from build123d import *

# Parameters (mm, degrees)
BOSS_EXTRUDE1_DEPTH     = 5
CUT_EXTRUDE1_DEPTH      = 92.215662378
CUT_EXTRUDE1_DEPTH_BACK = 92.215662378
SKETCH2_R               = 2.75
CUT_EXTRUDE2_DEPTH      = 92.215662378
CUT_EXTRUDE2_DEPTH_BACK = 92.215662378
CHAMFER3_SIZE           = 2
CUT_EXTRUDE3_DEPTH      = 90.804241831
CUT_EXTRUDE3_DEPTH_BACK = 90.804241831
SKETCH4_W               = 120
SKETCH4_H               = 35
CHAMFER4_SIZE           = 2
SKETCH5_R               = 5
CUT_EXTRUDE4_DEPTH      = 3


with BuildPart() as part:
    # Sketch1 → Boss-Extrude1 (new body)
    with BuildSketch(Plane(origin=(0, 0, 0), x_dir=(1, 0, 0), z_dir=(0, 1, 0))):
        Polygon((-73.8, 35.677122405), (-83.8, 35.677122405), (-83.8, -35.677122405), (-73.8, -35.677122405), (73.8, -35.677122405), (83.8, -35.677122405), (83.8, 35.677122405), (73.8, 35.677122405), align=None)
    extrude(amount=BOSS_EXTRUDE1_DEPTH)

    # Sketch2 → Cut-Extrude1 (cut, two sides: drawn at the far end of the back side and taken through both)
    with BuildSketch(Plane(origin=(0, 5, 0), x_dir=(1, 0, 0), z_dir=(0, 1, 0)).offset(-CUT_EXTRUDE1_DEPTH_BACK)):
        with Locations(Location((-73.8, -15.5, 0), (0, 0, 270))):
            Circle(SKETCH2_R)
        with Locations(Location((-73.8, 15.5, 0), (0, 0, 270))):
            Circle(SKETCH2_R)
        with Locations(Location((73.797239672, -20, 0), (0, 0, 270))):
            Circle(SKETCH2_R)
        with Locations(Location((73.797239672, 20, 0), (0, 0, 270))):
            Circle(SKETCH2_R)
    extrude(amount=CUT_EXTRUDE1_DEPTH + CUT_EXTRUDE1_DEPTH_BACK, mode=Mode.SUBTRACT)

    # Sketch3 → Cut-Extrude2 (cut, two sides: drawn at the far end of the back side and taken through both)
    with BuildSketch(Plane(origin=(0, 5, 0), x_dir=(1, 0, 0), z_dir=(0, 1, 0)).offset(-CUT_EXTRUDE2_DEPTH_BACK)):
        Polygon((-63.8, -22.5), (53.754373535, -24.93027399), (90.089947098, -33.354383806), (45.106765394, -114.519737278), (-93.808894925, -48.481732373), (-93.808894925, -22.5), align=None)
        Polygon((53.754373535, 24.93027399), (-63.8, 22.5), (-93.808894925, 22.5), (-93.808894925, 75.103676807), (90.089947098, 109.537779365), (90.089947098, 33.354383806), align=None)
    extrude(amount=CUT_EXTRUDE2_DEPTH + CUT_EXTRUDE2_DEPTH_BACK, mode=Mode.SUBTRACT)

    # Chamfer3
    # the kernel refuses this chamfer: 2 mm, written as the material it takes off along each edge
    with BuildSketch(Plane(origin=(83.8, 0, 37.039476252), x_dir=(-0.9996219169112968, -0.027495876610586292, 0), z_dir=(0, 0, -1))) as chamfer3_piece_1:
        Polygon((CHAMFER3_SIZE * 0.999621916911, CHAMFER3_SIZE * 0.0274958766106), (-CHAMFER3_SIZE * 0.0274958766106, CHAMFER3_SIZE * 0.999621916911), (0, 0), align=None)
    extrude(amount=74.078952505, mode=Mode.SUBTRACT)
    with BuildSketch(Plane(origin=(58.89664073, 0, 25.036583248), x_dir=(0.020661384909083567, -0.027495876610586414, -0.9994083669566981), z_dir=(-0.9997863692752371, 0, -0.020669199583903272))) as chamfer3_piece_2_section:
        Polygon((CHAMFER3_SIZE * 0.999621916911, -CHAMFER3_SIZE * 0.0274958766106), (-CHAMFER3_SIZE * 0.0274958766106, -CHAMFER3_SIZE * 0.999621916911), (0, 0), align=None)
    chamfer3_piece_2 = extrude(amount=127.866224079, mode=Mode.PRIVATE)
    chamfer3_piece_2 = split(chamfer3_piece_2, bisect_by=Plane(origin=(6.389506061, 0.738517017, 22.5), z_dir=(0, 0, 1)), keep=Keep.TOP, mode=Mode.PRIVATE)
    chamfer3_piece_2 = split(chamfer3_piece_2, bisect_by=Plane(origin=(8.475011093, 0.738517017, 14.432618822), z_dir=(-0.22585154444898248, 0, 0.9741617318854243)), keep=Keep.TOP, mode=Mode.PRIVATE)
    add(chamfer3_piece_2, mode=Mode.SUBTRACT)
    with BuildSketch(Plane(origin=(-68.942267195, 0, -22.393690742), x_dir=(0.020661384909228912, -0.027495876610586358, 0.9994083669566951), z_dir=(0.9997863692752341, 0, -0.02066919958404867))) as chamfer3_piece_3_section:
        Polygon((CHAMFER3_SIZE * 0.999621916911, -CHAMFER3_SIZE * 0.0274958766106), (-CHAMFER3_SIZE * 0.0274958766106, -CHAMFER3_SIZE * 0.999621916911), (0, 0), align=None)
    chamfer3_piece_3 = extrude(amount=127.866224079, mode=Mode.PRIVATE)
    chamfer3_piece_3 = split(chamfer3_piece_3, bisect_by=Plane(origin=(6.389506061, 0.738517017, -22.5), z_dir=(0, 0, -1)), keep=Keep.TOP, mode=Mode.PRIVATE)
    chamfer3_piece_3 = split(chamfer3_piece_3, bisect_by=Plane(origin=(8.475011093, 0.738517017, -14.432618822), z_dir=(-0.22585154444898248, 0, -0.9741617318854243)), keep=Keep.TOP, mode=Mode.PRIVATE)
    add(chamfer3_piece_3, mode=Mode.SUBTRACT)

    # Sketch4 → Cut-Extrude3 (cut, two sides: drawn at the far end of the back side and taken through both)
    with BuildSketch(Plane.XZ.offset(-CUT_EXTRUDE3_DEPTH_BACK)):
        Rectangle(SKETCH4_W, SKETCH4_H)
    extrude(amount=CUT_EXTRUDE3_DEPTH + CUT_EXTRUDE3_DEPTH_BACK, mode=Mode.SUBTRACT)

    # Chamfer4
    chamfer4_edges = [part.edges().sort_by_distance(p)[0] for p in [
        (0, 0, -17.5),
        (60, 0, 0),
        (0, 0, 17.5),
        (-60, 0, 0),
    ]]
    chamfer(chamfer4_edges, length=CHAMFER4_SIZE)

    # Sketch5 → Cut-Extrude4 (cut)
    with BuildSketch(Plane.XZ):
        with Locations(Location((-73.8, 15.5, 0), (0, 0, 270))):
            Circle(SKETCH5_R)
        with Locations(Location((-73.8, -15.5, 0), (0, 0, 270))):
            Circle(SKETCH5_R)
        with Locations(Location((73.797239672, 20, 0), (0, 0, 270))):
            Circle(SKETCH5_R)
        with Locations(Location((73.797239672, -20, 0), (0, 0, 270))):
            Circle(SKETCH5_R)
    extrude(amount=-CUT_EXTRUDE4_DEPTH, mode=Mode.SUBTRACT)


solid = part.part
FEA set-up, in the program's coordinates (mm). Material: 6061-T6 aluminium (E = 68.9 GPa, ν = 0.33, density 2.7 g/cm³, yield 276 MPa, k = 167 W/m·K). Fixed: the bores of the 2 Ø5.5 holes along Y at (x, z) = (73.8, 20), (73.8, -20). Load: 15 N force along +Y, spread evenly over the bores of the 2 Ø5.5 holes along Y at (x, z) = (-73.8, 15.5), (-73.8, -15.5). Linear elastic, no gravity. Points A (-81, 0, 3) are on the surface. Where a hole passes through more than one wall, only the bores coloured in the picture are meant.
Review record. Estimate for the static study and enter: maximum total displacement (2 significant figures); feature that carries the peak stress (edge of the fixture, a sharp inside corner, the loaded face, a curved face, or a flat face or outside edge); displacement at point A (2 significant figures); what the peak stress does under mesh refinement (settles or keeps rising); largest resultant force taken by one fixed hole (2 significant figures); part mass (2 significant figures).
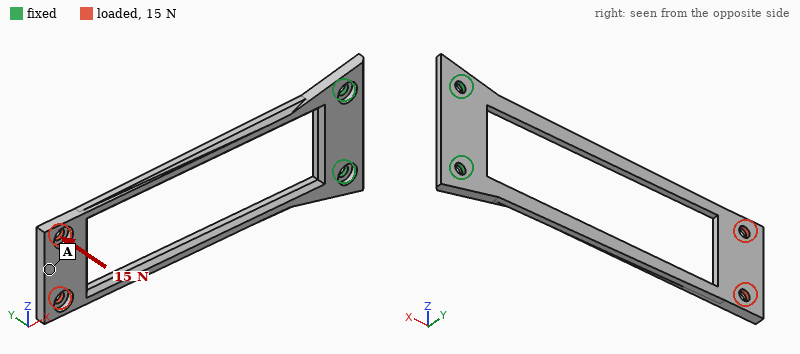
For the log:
2.0 mm
edge of the fixture
2.0 mm
keeps rising
12 N
48 g
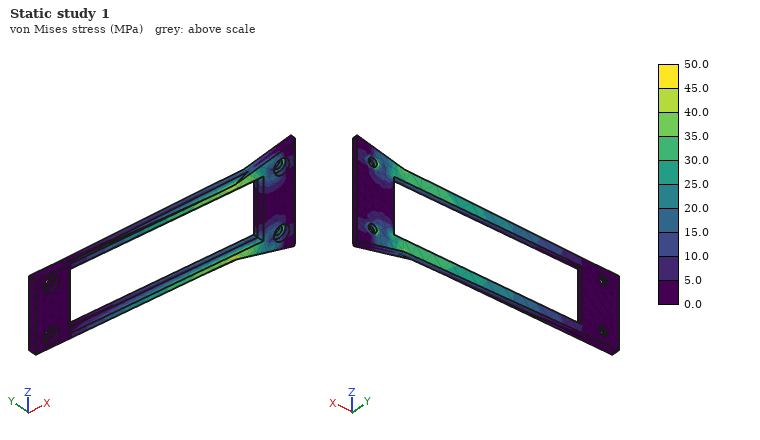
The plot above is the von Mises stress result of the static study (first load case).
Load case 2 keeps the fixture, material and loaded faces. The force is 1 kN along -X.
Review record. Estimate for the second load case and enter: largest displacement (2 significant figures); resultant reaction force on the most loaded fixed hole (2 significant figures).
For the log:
1.8 mm
500 N
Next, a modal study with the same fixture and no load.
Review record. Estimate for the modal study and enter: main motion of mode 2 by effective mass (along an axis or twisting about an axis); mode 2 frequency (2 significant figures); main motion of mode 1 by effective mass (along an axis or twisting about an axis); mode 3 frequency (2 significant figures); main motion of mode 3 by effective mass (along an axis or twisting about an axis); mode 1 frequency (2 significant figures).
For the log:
along Z
320 Hz
along Y
560 Hz
twisting about X
120 Hz
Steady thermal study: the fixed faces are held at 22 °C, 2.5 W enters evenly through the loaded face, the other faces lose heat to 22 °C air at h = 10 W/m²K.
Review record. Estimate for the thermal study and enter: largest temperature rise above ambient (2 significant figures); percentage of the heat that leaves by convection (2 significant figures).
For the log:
23 K
45 %
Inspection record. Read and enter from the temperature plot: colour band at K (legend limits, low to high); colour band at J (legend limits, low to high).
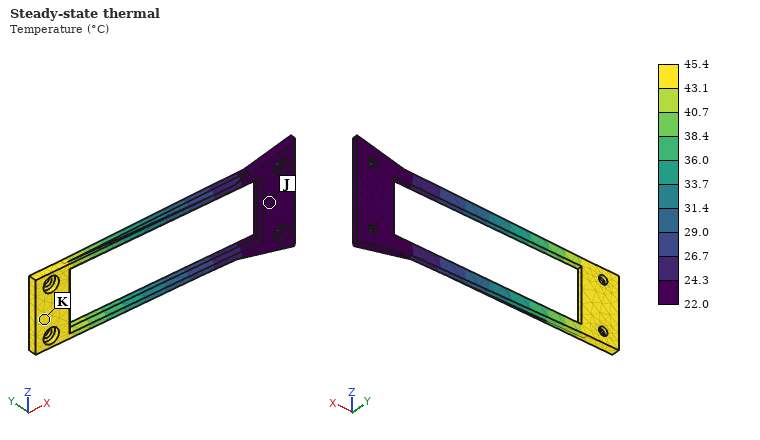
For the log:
43.1 to 45.4 °C
22.0 to 24.3 °C
